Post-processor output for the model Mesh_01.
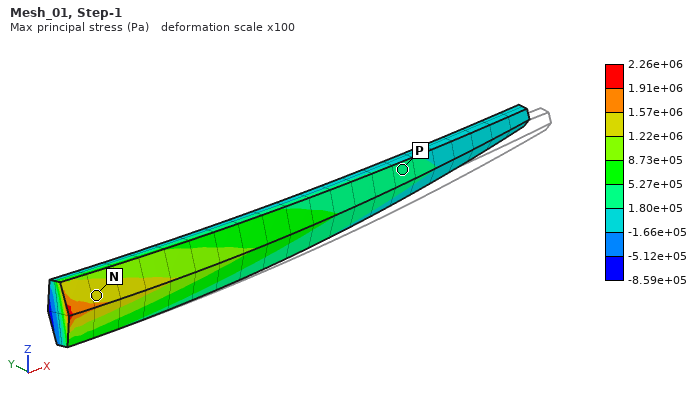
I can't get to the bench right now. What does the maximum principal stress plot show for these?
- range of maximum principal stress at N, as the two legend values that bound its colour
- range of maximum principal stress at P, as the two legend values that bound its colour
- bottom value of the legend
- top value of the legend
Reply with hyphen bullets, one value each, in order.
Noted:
- 1.22e+06 to 1.57e+06 Pa
- 1.80e+05 to 5.27e+05 Pa
- -8.59e+05 Pa
- 2.26e+06 Pa
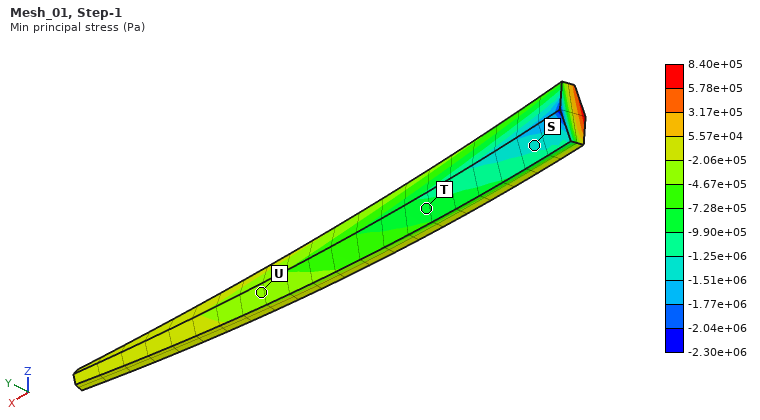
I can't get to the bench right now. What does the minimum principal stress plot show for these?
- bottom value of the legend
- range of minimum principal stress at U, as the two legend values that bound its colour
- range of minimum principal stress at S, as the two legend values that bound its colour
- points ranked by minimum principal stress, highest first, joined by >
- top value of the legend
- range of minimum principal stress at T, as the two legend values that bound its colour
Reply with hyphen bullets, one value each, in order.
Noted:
- -2.30e+06 Pa
- -4.67e+05 to -2.06e+05 Pa
- -1.51e+06 to -1.25e+06 Pa
- U > T > S
- 8.40e+05 Pa
- -9.90e+05 to -7.28e+05 Pa
